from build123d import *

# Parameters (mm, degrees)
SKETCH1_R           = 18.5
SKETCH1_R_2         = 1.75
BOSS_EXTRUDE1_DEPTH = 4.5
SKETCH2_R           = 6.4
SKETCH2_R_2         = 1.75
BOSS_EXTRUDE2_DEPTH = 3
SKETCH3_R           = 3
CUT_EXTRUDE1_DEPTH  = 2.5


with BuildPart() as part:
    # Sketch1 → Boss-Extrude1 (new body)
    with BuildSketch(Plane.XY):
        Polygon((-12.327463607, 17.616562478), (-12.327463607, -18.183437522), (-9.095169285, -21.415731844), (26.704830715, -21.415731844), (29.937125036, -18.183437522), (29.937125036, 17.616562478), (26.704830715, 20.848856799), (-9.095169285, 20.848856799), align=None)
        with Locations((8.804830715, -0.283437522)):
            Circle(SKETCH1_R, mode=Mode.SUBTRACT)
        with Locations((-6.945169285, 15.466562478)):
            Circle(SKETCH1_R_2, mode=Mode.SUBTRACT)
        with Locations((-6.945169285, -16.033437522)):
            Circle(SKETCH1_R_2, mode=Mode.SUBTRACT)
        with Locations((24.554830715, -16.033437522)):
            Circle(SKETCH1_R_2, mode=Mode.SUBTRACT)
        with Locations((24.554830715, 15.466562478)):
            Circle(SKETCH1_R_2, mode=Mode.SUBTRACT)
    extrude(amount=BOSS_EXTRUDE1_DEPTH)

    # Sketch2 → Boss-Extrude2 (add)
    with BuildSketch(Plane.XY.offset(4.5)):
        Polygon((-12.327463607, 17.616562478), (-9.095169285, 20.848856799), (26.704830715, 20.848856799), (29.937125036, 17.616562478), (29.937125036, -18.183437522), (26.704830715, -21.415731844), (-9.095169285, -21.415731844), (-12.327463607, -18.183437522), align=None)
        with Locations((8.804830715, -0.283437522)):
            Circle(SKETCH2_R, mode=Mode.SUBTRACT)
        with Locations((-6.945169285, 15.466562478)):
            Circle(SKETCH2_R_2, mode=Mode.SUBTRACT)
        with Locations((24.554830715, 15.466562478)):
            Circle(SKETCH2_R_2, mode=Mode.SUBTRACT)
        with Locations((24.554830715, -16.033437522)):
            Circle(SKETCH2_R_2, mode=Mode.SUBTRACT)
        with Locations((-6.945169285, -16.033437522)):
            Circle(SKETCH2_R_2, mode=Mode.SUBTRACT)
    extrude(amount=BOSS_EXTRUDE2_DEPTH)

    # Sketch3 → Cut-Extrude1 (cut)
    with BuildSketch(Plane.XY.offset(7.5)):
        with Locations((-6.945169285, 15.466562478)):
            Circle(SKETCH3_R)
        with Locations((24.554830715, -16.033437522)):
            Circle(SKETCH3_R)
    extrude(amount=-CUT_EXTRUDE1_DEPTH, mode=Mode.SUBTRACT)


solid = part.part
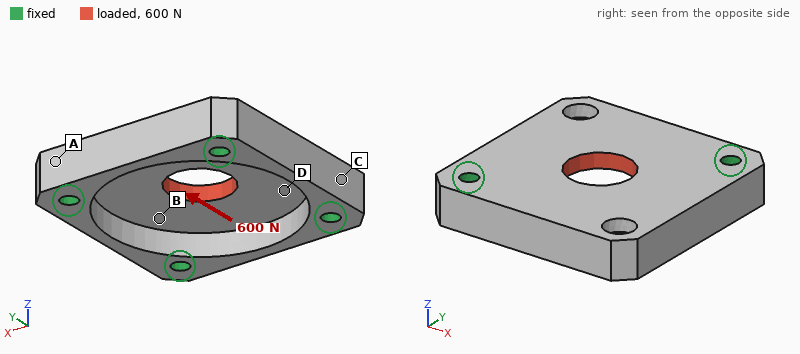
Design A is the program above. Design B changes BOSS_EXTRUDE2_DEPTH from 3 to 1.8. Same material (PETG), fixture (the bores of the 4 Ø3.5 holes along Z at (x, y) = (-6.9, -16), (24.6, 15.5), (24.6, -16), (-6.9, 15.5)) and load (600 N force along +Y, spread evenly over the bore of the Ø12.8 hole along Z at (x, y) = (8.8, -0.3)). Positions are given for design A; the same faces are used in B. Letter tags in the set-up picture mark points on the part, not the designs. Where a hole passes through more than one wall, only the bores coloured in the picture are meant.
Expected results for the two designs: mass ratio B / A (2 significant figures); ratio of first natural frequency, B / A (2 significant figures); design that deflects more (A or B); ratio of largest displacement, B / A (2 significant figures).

0.75
0.75
B
1.5
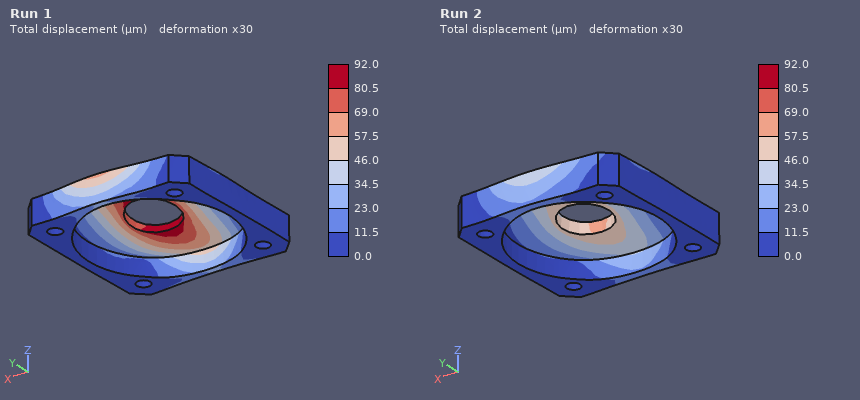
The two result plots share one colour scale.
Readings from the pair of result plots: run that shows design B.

Run 1
